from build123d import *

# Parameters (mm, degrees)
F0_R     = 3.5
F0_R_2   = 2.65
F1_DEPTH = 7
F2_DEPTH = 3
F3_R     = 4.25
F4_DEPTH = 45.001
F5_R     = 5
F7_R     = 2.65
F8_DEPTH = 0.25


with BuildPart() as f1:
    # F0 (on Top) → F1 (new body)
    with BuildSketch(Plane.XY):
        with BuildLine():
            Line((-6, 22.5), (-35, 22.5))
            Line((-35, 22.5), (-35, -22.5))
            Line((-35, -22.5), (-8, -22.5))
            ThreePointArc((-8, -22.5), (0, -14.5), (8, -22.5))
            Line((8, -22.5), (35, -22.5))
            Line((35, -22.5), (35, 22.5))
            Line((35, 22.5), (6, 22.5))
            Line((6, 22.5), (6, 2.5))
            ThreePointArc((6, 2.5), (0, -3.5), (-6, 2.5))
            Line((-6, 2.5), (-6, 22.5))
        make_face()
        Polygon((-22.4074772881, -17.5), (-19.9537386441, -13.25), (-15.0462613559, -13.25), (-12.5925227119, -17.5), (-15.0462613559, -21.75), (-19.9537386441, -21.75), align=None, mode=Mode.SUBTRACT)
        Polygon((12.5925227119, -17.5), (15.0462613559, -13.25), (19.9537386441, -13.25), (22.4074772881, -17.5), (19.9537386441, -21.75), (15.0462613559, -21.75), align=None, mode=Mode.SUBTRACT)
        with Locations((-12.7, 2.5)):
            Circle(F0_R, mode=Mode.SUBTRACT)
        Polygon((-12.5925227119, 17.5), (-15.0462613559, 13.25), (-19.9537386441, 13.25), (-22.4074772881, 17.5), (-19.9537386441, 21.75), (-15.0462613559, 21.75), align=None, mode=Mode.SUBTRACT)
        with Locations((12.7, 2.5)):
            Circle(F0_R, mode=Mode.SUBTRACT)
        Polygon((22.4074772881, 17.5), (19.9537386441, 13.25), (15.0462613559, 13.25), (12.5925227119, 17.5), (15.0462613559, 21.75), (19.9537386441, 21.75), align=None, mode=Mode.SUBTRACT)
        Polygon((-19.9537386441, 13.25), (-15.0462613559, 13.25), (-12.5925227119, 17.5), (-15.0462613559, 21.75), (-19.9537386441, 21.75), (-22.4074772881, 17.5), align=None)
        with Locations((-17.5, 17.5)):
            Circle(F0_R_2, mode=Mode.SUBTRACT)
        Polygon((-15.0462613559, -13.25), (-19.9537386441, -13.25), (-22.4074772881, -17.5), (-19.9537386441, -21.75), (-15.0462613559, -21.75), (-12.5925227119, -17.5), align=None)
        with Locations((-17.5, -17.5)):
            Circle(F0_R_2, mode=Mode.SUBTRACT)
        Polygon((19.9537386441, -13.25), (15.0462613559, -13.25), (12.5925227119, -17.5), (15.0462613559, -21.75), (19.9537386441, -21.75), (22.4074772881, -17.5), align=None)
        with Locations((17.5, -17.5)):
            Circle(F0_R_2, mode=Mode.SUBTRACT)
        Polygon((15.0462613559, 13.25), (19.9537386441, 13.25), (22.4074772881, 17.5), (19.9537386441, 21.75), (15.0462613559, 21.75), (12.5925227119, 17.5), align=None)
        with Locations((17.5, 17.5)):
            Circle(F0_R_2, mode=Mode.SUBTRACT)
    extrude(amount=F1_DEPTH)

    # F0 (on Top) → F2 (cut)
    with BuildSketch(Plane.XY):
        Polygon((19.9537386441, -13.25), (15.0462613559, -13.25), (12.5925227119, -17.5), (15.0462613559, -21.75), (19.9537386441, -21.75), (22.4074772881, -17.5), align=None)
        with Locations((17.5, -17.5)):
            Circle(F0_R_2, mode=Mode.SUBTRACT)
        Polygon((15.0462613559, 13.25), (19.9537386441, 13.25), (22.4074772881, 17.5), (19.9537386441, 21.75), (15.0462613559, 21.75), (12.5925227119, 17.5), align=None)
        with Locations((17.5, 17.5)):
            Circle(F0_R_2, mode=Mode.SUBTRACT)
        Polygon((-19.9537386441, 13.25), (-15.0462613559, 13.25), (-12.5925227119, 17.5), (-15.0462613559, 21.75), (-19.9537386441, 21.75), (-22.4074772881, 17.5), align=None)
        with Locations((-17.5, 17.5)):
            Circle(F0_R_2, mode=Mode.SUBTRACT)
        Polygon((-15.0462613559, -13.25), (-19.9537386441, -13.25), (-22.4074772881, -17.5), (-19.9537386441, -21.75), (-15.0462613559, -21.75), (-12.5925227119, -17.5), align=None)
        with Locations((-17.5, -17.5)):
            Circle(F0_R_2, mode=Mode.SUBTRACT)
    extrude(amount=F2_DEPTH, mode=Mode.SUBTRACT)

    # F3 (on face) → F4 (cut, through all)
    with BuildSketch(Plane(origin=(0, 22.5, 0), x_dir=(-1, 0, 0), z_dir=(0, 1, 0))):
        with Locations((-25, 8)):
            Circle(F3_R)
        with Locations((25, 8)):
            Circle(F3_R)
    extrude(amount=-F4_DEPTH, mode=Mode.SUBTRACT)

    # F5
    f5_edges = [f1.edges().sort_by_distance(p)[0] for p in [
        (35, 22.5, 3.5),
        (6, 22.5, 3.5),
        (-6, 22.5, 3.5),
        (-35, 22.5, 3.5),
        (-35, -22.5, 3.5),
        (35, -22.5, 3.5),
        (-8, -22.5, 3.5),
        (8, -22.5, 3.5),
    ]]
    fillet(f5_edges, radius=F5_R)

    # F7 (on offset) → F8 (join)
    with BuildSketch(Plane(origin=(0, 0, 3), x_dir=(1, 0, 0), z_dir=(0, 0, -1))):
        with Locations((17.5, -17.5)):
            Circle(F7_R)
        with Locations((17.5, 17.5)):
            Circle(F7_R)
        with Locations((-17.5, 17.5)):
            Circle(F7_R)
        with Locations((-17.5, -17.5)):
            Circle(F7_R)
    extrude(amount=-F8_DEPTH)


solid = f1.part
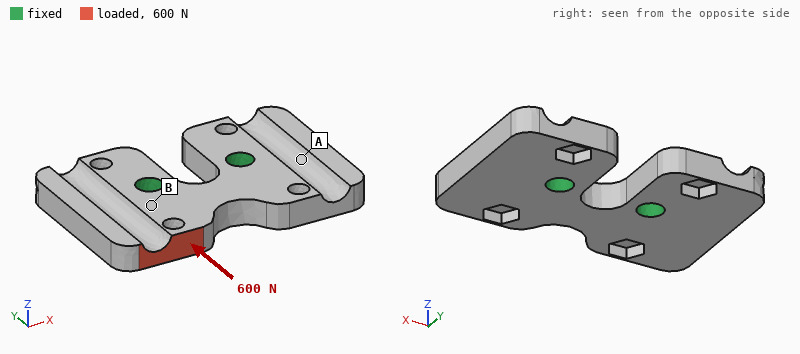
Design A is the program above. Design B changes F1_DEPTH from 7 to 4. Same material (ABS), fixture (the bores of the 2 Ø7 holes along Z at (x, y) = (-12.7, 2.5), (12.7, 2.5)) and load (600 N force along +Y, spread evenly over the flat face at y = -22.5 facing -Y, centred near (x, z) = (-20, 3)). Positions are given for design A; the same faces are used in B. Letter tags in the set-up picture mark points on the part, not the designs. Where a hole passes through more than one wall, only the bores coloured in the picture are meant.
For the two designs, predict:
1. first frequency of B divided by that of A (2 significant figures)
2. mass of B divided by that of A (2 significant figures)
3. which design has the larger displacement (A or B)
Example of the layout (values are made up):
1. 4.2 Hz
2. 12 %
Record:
1. 0.68
2. 0.62
3. B
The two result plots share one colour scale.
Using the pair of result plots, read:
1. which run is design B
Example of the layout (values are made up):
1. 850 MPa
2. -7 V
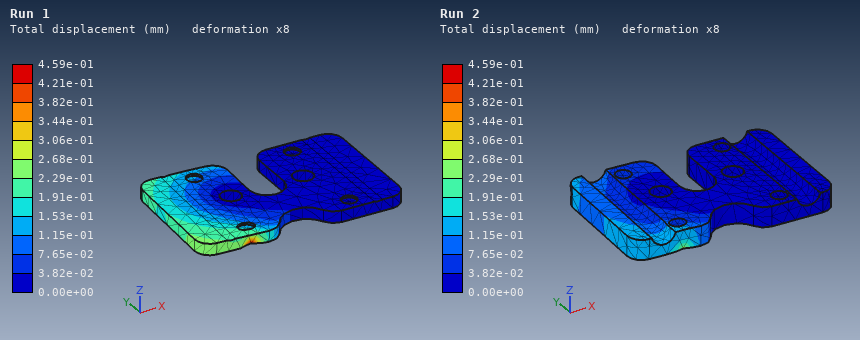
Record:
1. Run 1
